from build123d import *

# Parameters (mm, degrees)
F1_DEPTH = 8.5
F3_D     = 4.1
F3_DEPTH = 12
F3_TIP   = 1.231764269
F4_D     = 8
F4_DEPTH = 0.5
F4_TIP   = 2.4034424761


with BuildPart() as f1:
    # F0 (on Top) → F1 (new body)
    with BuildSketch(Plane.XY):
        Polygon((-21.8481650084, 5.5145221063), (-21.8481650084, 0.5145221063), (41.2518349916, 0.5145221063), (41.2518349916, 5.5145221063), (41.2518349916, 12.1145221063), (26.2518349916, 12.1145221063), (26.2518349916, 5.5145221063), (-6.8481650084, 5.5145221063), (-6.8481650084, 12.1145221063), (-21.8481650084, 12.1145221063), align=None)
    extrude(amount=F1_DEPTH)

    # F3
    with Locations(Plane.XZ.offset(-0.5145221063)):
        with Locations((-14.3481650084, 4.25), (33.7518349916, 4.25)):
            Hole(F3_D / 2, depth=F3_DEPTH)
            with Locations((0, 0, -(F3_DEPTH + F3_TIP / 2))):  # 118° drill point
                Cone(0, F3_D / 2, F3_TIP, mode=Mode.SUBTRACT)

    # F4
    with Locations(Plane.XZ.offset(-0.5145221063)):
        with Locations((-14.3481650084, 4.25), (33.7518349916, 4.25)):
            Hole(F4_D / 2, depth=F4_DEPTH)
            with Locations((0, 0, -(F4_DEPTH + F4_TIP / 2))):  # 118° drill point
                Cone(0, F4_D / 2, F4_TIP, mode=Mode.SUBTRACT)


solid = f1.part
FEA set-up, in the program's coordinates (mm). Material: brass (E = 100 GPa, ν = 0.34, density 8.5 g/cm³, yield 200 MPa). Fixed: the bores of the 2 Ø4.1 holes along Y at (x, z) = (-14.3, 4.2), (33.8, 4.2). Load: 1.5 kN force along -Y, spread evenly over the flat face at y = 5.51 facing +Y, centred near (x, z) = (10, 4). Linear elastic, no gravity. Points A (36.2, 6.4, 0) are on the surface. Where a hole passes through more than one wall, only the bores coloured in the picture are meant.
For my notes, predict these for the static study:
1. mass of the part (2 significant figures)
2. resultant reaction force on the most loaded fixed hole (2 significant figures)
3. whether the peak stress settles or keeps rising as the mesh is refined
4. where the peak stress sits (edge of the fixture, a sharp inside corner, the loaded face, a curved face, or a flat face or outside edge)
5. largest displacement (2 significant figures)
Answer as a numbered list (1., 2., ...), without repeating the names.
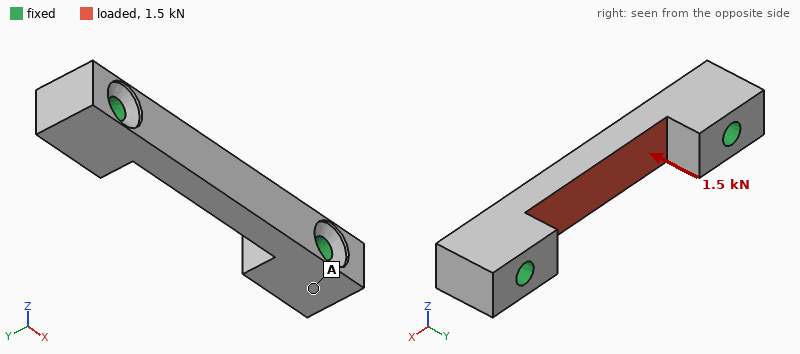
1. 34 g
2. 830 N
3. keeps rising
4. edge of the fixture
5. 37 µm
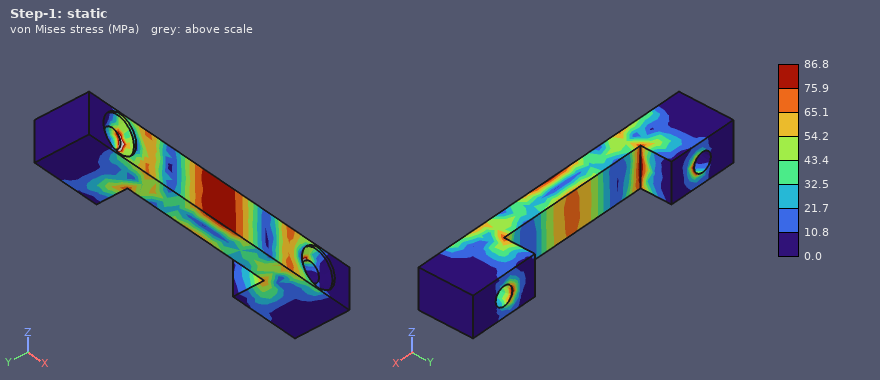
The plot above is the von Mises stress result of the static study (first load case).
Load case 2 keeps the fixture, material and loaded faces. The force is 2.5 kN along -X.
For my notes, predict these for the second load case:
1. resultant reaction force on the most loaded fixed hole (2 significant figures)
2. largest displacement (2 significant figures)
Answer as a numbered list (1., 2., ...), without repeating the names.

1. 1.3 kN
2. 5.8 µm
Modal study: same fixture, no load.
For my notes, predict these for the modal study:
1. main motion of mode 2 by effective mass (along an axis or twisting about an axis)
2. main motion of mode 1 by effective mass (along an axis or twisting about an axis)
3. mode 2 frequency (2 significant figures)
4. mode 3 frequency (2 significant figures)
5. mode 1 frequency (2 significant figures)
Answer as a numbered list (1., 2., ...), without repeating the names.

1. along Z
2. along Y
3. 12 kHz
4. 23 kHz
5. 11 kHz
